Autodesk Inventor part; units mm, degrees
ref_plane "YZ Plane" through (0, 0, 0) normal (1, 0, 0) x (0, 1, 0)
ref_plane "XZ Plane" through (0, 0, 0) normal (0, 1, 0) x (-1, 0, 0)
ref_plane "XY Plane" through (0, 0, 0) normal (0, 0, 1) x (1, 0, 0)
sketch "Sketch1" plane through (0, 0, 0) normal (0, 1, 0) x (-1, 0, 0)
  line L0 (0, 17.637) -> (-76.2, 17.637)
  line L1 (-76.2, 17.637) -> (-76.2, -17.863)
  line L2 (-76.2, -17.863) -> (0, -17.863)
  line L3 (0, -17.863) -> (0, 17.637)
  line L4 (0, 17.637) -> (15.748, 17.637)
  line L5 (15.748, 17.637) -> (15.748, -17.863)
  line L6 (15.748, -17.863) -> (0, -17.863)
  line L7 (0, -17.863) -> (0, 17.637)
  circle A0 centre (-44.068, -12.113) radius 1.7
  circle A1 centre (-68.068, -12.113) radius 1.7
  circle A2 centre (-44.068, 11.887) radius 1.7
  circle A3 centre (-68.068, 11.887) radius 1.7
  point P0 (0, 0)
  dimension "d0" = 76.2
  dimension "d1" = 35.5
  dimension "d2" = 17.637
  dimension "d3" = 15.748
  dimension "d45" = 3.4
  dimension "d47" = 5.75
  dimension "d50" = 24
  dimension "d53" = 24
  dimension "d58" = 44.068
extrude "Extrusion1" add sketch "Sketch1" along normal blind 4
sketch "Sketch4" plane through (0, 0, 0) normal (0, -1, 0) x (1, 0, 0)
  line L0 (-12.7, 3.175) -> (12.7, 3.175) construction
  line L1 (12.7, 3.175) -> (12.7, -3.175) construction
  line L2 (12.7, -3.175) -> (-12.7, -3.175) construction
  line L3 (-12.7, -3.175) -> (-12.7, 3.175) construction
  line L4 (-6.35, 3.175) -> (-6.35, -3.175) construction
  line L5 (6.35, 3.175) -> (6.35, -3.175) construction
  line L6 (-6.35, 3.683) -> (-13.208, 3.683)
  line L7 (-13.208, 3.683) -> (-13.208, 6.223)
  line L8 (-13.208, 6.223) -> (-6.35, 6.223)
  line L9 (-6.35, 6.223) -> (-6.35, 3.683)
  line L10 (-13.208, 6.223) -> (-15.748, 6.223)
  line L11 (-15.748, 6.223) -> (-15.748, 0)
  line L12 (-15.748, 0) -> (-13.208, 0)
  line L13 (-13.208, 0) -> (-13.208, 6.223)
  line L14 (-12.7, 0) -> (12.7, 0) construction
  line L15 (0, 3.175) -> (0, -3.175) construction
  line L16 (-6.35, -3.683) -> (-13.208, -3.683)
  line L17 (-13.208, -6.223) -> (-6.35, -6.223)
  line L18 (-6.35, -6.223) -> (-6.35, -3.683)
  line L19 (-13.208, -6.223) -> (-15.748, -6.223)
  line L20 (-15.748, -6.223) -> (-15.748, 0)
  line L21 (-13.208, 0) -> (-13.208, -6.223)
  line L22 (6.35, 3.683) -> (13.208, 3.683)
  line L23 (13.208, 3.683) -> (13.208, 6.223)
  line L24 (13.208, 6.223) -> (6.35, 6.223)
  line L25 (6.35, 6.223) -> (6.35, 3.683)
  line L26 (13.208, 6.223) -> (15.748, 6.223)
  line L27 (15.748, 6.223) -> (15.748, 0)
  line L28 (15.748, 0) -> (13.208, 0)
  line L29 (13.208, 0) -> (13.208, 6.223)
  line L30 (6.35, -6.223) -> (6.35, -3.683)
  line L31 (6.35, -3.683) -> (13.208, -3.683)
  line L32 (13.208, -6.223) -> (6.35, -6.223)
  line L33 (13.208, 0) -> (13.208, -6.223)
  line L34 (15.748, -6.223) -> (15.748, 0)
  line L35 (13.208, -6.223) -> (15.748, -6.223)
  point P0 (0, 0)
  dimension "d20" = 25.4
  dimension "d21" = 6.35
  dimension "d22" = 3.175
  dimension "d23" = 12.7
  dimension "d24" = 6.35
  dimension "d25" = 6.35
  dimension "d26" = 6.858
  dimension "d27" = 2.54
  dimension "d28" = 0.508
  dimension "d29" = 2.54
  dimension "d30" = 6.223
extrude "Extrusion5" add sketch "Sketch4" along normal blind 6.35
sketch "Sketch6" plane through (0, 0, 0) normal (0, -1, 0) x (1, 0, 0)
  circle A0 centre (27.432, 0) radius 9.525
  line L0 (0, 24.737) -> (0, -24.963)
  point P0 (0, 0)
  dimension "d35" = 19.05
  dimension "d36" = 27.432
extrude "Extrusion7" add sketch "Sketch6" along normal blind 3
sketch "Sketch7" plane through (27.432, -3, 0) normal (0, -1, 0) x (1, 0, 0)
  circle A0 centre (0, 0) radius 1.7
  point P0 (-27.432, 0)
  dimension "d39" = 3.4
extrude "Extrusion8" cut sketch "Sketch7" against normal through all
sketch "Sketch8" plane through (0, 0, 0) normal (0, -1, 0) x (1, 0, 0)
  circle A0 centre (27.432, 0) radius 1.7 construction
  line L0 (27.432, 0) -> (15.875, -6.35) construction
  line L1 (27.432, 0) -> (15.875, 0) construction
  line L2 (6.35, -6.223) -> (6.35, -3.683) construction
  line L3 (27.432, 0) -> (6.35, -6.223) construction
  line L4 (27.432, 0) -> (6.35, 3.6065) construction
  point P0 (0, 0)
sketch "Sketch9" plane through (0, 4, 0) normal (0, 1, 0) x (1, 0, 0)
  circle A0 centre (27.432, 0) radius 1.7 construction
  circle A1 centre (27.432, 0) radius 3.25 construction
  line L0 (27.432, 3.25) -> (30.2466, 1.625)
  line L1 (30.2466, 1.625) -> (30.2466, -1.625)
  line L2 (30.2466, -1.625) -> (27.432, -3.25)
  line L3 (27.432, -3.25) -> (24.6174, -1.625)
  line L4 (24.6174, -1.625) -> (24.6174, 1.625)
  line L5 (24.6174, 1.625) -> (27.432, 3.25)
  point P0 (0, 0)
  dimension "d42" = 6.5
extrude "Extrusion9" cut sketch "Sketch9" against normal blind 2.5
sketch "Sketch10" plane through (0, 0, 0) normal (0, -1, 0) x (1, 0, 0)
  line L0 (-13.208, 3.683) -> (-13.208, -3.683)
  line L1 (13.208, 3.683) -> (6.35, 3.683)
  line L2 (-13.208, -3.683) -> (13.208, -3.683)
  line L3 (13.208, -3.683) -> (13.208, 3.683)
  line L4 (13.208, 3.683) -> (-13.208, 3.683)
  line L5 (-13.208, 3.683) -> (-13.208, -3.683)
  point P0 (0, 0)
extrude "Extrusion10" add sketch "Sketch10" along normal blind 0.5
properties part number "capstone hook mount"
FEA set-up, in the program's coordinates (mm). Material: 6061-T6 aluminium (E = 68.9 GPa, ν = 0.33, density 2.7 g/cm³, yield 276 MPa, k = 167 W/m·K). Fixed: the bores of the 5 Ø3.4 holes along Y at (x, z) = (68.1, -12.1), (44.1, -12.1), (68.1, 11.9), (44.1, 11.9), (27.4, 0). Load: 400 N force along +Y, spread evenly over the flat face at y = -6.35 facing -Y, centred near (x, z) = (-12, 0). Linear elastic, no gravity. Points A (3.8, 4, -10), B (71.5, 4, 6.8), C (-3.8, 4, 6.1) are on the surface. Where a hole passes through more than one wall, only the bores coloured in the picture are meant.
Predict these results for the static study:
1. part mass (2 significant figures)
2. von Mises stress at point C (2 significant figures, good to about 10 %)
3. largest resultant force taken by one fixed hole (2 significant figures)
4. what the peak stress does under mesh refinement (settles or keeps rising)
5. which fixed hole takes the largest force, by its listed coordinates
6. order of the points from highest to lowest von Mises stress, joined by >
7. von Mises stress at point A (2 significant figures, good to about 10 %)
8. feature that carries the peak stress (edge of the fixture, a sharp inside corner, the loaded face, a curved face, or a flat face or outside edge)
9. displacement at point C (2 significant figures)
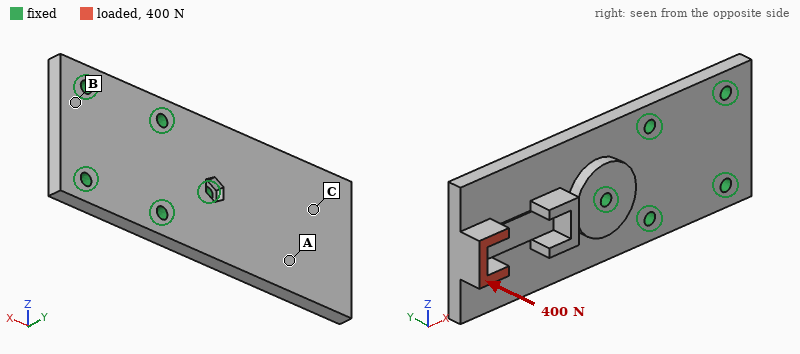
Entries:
39 g
33 MPa
1.4 kN
keeps rising
(27.4, 0)
A > C > B
60 MPa
edge of the fixture
0.30 mm
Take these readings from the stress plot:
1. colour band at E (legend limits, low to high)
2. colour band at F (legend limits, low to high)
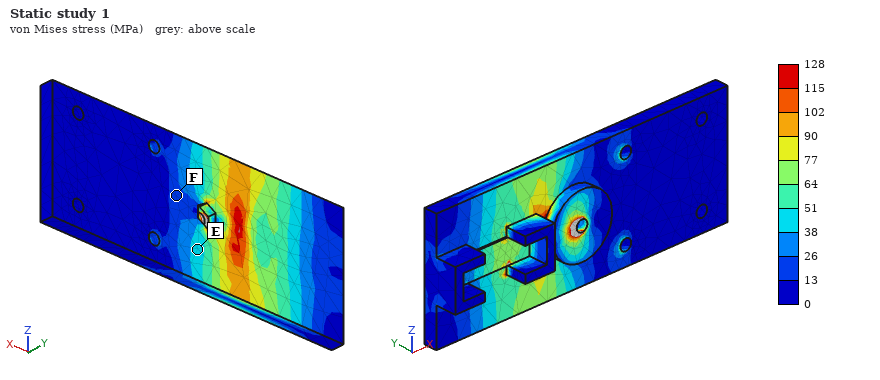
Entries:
38 to 51 MPa
13 to 26 MPa
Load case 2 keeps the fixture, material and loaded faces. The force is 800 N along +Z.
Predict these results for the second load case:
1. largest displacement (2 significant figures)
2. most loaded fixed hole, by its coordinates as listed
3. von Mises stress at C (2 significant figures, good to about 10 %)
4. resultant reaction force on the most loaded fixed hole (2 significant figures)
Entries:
0.19 mm
(27.4, 0)
44 MPa
1.4 kN
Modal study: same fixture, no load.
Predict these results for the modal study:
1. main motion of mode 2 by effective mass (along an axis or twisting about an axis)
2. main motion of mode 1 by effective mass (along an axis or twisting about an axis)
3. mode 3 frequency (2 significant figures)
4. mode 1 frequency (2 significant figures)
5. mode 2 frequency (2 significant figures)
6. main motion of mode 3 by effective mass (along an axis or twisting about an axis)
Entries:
twisting about X
along Y
7300 Hz
1900 Hz
4400 Hz
along Z
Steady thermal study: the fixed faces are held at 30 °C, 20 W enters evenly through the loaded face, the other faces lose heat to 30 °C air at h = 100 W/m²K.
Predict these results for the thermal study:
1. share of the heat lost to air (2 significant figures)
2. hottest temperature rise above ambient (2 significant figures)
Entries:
34 %
39 K
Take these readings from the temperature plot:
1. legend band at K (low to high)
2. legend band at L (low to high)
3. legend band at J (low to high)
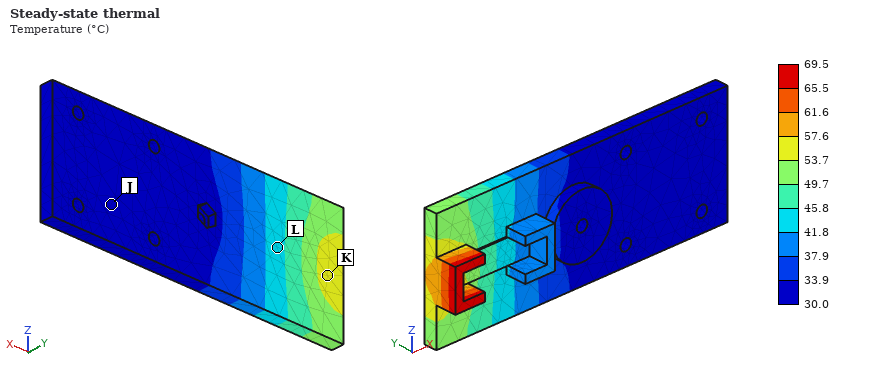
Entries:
53.7 to 57.6 °C
41.8 to 45.8 °C
30.0 to 33.9 °C
